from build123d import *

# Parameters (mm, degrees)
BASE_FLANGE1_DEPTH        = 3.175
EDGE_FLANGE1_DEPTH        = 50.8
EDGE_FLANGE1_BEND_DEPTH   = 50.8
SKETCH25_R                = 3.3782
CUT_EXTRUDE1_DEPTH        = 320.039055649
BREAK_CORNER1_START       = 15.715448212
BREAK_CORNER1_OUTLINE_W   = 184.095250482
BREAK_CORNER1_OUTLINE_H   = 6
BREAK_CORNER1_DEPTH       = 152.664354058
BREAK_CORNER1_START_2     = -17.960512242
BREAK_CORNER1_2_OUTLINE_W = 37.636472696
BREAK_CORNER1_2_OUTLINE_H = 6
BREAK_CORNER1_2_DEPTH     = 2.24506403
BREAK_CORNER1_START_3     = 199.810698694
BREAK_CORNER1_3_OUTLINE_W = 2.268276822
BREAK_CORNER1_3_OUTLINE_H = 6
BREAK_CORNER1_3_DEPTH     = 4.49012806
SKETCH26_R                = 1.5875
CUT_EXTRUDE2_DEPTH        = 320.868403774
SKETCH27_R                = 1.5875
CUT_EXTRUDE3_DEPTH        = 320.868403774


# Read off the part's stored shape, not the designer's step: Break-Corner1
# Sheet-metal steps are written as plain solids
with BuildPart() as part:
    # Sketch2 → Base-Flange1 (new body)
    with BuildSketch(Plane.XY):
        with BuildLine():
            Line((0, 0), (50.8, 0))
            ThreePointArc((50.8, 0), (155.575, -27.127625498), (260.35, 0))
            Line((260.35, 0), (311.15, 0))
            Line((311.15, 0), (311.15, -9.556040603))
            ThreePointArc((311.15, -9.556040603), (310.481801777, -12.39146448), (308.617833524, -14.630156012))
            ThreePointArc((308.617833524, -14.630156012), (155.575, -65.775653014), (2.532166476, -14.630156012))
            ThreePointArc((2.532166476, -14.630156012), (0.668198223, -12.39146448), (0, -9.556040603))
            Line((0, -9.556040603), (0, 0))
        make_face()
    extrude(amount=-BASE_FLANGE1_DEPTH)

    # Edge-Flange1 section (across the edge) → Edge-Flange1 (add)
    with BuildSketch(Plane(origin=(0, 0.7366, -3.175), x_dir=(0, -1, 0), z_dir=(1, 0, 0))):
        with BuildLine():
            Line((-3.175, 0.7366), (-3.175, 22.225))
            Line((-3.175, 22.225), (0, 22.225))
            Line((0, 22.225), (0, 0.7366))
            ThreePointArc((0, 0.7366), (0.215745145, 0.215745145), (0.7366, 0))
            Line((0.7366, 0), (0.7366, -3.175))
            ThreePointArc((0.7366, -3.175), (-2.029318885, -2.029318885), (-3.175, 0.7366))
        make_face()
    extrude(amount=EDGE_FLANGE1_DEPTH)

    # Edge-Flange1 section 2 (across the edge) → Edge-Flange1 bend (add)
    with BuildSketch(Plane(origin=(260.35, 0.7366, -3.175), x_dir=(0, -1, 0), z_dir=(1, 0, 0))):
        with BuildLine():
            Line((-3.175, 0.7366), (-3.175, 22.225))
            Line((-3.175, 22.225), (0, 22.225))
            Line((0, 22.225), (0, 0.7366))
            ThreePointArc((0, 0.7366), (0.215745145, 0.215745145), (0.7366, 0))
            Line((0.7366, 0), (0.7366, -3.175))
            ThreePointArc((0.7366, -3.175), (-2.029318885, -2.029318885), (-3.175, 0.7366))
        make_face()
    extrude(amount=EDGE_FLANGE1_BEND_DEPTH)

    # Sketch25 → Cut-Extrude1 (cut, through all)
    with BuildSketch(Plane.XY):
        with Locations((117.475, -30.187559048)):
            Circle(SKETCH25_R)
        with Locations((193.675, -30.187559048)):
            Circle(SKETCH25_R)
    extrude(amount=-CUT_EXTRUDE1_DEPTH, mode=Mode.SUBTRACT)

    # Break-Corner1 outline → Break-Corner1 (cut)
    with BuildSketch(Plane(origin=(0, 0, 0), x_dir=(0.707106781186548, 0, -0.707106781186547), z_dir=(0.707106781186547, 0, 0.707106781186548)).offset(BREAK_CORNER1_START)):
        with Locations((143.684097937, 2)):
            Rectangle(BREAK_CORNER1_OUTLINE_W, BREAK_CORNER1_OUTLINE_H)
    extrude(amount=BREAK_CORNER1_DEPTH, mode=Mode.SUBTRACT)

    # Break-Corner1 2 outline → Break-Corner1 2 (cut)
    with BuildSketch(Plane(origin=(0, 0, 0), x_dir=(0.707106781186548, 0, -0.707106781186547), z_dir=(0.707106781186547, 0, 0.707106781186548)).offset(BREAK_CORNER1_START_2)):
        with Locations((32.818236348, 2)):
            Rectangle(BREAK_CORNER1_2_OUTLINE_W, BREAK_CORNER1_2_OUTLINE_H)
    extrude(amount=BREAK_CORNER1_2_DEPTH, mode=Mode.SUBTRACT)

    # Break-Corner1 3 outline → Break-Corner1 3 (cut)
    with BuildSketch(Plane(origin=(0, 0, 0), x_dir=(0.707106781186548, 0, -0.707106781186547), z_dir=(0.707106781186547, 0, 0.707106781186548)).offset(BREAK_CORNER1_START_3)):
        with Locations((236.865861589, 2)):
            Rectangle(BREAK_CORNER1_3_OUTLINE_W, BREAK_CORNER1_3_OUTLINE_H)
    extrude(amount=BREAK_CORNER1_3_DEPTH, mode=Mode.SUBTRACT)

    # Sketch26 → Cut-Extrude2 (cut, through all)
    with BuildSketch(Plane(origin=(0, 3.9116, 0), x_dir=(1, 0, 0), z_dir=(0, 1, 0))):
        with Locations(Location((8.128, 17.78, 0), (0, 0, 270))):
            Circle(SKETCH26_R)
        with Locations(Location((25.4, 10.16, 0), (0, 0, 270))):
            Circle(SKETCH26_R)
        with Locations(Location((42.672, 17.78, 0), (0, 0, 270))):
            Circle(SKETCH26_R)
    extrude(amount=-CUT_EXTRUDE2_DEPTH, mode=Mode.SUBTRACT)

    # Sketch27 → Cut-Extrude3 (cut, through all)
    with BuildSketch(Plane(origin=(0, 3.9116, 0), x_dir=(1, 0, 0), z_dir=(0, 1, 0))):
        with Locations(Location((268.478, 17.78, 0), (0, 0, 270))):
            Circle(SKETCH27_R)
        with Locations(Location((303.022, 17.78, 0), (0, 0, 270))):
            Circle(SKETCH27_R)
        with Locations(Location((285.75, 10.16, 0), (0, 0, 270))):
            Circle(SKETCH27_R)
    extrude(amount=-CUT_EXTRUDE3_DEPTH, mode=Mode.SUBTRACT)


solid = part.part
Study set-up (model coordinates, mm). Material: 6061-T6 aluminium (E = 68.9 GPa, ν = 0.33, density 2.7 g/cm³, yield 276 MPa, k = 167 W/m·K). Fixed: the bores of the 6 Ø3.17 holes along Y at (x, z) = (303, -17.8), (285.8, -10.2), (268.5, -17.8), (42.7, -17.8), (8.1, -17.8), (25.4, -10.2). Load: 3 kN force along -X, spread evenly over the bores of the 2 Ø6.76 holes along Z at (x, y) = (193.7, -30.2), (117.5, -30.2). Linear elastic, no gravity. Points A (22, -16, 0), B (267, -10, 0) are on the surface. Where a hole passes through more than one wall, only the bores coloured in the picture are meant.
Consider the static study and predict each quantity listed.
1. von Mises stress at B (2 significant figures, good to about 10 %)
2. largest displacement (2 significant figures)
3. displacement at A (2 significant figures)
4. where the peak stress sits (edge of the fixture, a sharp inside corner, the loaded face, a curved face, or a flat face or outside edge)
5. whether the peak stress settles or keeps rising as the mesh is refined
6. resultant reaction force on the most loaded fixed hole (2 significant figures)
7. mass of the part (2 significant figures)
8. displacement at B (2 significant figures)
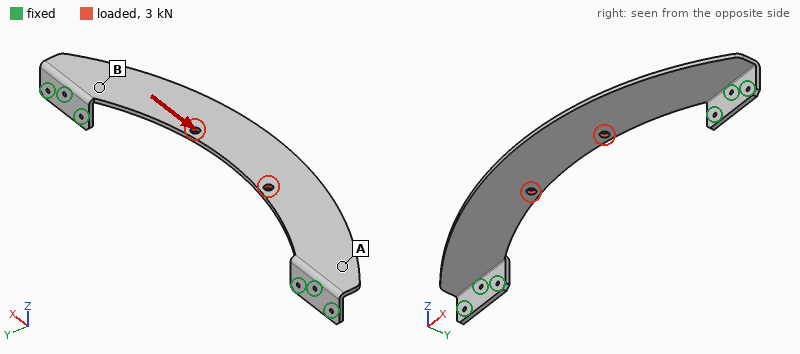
24 MPa
94 µm
56 µm
edge of the fixture
keeps rising
1.1 kN
120 g
33 µm
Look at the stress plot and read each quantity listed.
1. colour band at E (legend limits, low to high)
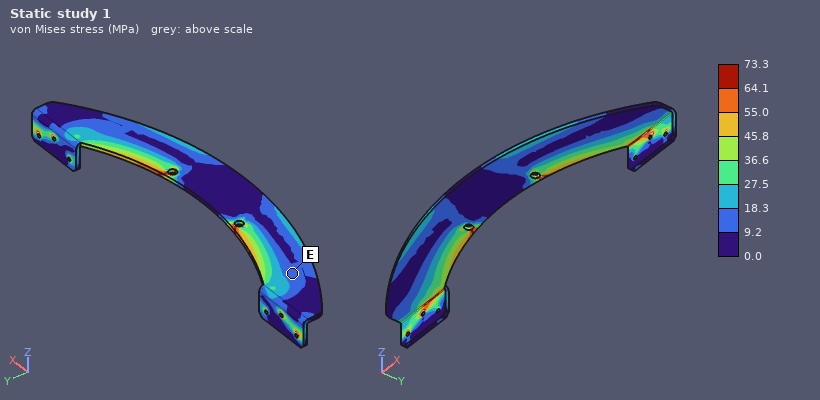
9.2 to 18.3 MPa
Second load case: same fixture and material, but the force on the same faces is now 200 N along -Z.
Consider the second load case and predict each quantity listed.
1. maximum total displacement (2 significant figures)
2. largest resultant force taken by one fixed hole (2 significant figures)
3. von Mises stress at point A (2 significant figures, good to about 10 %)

2.5 mm
360 N
36 MPa
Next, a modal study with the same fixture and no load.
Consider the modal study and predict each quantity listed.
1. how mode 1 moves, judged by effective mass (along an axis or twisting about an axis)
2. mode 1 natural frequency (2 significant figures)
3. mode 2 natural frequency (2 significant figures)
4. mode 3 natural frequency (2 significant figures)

along Z
210 Hz
560 Hz
890 Hz
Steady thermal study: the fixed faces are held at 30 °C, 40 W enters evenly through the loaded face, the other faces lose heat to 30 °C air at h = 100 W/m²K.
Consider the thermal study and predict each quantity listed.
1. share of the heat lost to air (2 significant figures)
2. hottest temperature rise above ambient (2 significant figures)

87 %
40 K
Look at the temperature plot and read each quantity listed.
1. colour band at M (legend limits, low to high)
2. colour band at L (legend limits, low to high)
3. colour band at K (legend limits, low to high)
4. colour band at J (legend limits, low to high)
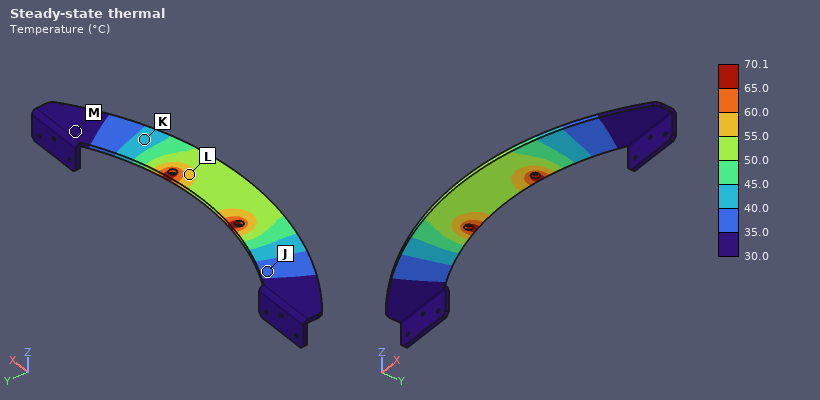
30.0 to 35.0 °C
55.0 to 60.0 °C
40.0 to 45.0 °C
35.0 to 40.0 °C
